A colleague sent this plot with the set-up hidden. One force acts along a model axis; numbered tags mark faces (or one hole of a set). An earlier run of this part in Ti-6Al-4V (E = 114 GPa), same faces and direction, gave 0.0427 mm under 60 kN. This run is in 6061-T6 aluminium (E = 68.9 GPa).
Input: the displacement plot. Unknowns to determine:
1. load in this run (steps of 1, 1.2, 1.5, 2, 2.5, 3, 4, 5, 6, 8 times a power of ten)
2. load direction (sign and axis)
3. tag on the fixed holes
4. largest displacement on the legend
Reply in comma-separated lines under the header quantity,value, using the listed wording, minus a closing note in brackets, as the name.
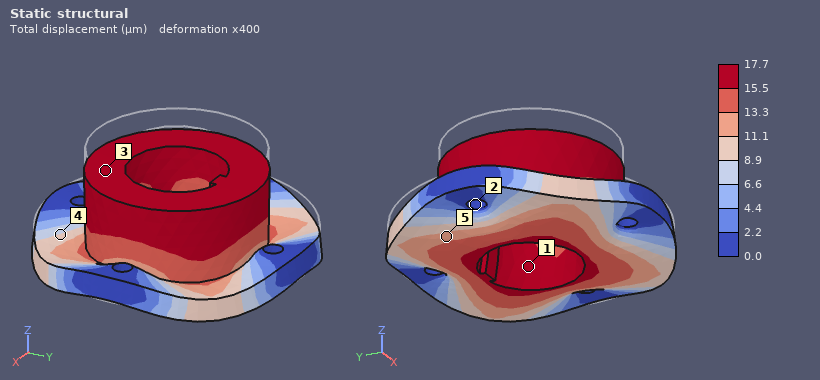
quantity,value
load in this run,15 kN
load direction,-Z
tag on the fixed holes,2
largest displacement on the legend,17.7 µm
